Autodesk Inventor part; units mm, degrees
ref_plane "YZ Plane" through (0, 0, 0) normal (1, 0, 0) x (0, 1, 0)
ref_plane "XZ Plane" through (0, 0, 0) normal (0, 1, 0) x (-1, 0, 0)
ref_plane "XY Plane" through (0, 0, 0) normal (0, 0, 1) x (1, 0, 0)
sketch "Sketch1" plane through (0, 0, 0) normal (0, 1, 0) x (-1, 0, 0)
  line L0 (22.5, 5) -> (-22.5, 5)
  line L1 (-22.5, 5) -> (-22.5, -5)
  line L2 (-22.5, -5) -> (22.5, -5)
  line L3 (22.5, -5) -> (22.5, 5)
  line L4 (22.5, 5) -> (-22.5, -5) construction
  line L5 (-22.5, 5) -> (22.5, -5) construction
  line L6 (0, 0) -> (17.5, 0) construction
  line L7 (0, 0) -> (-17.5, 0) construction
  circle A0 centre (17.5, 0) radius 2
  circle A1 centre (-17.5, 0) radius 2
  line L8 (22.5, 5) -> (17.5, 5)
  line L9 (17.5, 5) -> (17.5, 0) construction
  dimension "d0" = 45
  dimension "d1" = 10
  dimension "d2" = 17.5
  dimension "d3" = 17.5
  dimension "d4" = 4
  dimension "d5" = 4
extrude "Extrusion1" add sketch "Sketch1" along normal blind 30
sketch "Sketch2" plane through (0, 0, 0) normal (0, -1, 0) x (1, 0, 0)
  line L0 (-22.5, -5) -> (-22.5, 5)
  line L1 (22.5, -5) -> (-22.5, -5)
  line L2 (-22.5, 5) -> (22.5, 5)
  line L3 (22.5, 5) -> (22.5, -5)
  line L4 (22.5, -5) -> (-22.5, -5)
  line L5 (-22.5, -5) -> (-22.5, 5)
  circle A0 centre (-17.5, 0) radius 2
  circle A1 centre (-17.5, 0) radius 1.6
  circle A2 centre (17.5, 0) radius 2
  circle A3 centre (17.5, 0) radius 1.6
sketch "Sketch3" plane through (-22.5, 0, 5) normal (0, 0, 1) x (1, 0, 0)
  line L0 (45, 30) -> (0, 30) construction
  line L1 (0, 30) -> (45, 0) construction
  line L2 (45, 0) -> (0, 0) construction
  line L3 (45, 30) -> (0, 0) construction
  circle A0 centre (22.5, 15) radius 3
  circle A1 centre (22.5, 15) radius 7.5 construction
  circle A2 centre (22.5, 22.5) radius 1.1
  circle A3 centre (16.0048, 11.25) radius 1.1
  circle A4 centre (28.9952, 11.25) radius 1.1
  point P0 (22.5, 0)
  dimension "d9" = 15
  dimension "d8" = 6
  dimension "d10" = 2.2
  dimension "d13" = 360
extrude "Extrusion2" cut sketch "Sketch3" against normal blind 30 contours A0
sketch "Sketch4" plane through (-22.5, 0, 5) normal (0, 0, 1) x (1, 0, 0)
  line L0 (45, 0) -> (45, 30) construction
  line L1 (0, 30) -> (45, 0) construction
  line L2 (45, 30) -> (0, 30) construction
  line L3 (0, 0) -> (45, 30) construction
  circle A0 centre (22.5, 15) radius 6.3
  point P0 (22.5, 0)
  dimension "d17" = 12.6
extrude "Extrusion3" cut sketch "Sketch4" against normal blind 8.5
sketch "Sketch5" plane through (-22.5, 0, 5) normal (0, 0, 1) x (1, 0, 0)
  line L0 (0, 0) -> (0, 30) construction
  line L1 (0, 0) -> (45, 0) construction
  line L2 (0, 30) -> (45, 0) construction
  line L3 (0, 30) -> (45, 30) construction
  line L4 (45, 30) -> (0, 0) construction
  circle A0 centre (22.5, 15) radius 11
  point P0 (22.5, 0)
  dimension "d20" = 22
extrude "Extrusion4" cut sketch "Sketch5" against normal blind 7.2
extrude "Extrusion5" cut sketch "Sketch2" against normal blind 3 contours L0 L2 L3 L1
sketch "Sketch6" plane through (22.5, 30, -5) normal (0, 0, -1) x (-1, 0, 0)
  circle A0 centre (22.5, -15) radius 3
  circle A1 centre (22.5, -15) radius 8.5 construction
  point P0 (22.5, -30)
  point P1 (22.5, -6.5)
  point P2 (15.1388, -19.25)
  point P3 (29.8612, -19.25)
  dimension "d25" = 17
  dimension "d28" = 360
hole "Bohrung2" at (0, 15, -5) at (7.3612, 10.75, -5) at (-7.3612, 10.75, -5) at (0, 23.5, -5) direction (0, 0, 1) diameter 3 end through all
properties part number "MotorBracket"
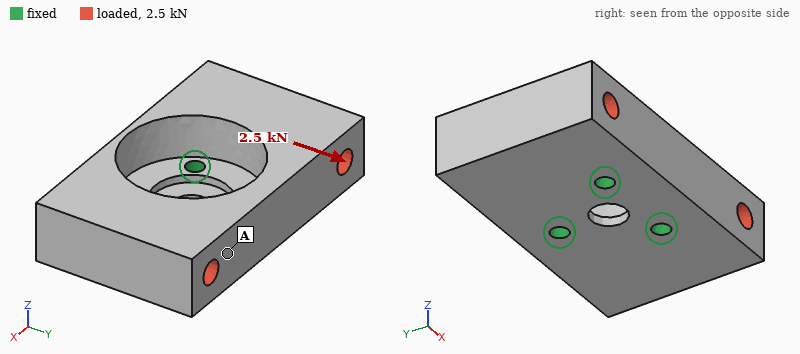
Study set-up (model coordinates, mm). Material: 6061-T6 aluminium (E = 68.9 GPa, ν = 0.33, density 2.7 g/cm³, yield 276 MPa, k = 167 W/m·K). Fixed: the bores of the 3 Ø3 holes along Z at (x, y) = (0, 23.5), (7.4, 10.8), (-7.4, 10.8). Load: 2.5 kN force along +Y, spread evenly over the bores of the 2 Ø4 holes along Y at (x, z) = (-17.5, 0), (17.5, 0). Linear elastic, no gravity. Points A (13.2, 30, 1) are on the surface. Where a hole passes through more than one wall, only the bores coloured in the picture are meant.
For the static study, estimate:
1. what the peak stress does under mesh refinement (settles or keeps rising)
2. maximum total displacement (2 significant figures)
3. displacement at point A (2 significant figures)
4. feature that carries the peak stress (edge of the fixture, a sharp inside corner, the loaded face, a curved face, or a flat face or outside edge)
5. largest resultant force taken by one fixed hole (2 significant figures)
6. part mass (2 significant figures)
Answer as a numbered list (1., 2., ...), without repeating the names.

1. keeps rising
2. 22 µm
3. 16 µm
4. edge of the fixture
5. 1.1 kN
6. 23 g
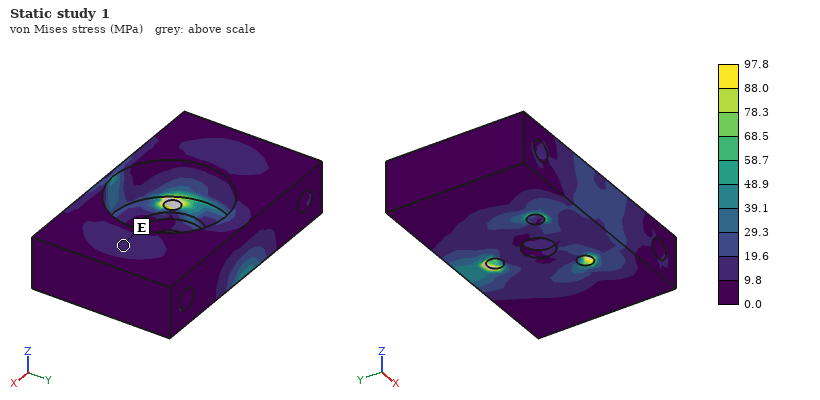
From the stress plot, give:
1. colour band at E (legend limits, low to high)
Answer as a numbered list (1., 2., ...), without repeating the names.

1. 9.8 to 19.6 MPa
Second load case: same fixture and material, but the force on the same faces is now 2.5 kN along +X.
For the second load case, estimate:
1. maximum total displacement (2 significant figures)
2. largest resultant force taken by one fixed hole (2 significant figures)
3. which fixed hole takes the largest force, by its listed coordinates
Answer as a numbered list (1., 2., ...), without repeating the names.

1. 34 µm
2. 1.2 kN
3. (0, 23.5)
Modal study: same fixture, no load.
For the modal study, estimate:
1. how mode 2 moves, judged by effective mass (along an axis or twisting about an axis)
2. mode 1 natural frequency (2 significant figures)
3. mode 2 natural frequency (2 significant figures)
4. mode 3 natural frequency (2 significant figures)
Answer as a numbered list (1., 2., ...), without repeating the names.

1. along Z
2. 7200 Hz
3. 11 kHz
4. 14 kHz
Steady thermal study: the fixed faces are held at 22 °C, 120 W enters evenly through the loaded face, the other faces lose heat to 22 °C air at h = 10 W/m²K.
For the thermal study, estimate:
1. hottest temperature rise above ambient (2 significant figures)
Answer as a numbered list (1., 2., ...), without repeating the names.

1. 43 K
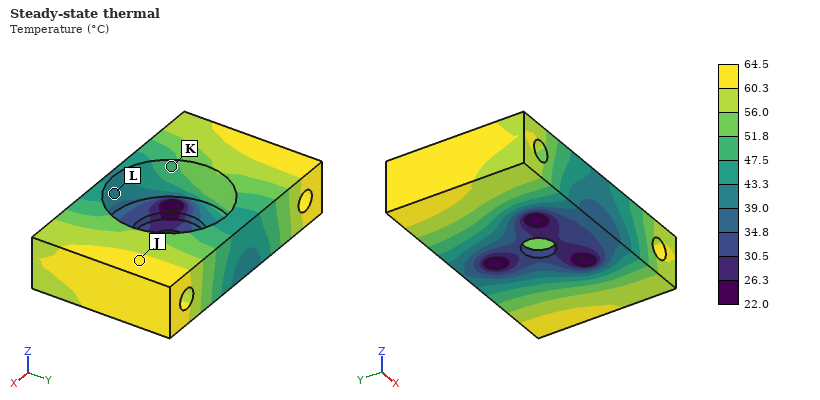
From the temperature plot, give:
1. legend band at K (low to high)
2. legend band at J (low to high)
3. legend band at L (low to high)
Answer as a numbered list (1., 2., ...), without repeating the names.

1. 47.5 to 51.8 °C
2. 60.3 to 64.5 °C
3. 39.0 to 43.3 °C
